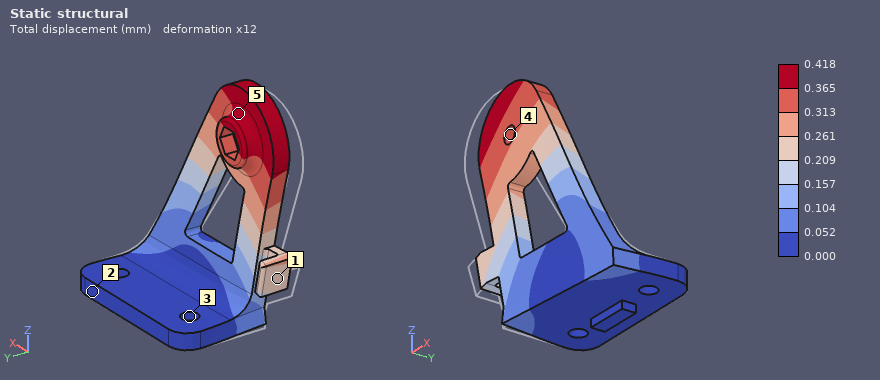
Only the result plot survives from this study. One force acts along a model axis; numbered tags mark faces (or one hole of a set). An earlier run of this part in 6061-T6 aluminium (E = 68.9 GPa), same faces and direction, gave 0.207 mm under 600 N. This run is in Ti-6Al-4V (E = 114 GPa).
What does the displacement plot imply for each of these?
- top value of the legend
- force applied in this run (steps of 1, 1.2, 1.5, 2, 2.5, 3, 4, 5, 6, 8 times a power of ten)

0.418 mm
2 kN
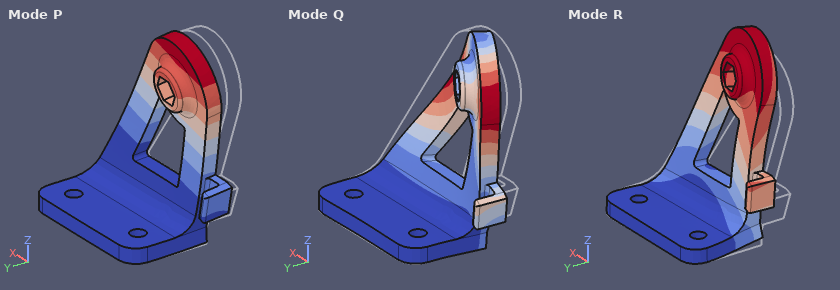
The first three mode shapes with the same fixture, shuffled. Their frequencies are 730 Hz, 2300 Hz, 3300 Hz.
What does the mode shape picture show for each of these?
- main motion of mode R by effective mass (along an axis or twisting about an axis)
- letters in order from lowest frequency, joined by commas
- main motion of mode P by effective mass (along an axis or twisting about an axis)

along X
P, R, Q
along Y
